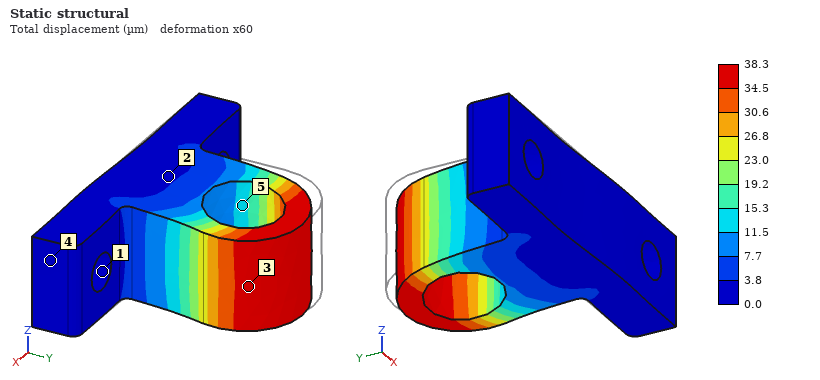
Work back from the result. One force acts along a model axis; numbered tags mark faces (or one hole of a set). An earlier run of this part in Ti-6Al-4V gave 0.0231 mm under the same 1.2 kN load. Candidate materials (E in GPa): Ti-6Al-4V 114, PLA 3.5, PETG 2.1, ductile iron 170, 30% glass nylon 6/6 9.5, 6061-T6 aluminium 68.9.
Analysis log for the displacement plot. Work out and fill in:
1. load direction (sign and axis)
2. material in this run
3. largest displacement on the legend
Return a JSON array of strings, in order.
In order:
["+X", "6061-T6 aluminium", "38.3 µm"]
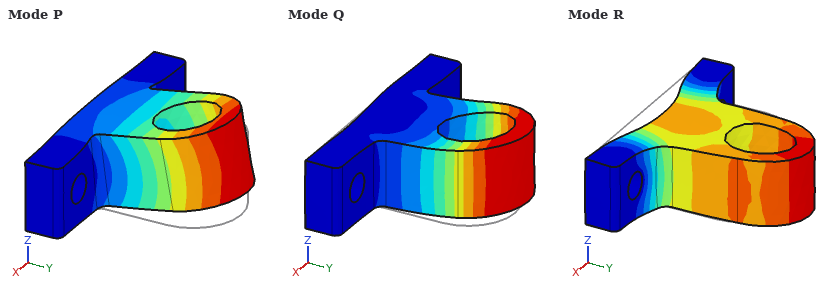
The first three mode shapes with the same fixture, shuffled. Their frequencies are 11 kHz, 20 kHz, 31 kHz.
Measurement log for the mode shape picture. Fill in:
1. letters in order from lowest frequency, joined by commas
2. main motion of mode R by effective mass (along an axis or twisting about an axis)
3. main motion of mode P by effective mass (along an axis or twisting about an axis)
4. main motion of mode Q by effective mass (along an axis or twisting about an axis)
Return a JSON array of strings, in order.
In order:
["P, Q, R", "along Y", "along Z", "along X"]
